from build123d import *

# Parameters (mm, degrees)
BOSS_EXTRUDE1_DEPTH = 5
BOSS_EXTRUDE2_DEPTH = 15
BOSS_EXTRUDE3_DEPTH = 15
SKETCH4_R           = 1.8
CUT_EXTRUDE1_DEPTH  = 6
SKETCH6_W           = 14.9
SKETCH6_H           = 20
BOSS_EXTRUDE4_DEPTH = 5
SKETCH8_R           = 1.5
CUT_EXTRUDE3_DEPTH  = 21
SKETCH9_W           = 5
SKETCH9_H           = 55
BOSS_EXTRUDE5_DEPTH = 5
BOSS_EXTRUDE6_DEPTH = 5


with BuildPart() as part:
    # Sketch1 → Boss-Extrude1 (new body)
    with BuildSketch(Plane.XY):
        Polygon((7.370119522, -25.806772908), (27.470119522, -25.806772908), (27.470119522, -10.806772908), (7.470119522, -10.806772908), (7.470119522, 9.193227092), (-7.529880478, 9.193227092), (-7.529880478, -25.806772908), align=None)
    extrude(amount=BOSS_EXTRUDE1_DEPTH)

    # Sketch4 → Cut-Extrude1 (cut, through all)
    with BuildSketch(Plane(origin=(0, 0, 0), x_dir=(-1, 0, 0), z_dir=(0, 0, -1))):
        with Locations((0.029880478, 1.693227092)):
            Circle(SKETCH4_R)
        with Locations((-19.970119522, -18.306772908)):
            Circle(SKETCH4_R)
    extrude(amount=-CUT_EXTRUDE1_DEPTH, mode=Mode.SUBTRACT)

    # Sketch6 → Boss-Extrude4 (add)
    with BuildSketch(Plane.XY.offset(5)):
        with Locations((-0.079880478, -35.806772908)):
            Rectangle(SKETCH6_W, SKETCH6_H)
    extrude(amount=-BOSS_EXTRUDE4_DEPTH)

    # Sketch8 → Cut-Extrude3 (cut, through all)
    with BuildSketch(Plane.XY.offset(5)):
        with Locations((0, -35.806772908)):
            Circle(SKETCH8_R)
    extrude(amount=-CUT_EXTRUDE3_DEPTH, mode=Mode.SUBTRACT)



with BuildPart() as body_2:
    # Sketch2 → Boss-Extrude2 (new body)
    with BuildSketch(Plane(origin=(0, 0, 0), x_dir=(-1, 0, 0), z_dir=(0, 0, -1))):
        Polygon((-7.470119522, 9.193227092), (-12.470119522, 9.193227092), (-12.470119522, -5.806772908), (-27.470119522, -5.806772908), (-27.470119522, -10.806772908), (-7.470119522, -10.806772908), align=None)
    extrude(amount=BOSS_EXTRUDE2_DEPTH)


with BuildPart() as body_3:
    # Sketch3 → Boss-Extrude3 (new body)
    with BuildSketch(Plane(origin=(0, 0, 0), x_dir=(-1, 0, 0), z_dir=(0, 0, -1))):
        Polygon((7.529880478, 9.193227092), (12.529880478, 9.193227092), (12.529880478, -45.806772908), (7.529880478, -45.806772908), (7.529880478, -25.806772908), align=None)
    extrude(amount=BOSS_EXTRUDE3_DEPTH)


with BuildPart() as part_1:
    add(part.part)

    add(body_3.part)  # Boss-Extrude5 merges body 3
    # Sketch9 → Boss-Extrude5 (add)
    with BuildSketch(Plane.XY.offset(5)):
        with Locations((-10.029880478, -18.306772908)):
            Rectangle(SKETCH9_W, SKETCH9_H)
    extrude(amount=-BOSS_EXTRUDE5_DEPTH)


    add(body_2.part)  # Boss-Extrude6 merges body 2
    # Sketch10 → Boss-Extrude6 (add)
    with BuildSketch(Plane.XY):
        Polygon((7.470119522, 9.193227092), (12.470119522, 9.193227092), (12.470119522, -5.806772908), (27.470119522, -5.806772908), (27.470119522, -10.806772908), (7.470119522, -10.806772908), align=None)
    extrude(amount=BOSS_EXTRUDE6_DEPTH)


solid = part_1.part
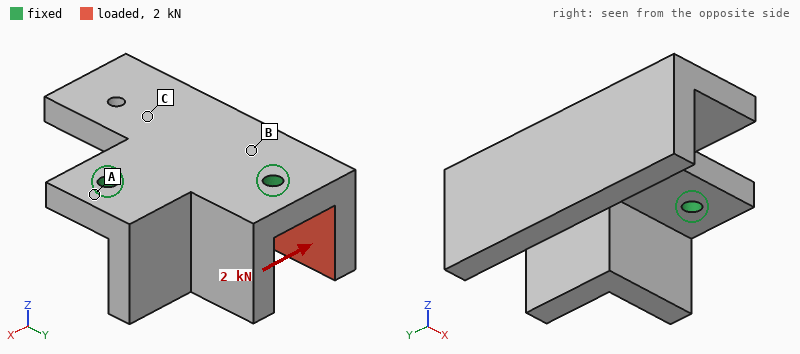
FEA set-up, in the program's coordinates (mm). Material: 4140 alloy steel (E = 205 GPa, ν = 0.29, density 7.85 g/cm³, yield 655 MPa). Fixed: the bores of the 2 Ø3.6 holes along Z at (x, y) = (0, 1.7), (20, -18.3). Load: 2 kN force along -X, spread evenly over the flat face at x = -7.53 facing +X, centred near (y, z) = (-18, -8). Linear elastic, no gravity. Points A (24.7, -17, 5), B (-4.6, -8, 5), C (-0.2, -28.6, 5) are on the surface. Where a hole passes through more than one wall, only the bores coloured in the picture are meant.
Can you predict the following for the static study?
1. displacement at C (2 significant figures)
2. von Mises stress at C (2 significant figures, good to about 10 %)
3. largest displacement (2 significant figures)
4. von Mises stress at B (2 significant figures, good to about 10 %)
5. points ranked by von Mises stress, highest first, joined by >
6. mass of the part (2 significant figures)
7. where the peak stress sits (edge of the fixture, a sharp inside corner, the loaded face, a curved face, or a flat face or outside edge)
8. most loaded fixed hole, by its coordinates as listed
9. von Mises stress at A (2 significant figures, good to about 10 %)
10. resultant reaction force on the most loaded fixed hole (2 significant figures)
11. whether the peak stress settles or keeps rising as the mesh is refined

0.020 mm
55 MPa
0.12 mm
93 MPa
B > C > A
110 g
edge of the fixture
(20, -18.3)
21 MPa
1.7 kN
keeps rising
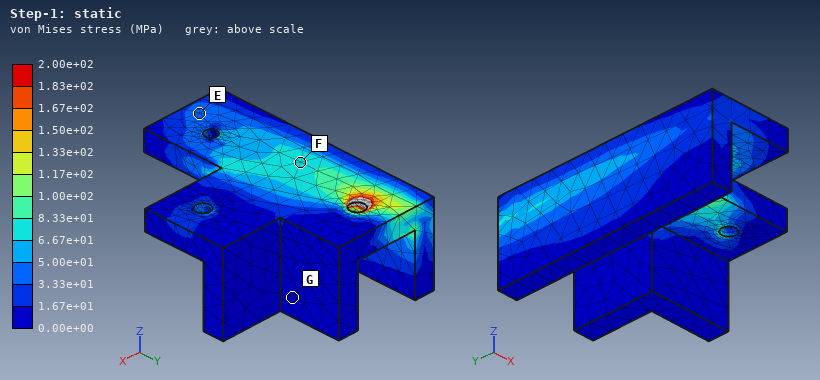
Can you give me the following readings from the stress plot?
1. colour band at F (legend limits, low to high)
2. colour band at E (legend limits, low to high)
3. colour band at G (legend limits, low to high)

6.67e+01 to 8.33e+01 MPa
3.33e+01 to 5.00e+01 MPa
0.00e+00 to 1.67e+01 MPa
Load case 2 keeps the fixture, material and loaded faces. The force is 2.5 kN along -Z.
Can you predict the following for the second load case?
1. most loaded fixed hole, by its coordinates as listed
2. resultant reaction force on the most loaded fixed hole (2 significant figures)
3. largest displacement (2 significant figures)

(0, 1.7)
1.8 kN
0.25 mm
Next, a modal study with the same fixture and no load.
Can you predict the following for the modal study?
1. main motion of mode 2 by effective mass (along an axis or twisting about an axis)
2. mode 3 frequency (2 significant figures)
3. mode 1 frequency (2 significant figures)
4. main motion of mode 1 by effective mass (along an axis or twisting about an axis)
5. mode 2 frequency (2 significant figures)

along X
8900 Hz
2400 Hz
along Z
5900 Hz
